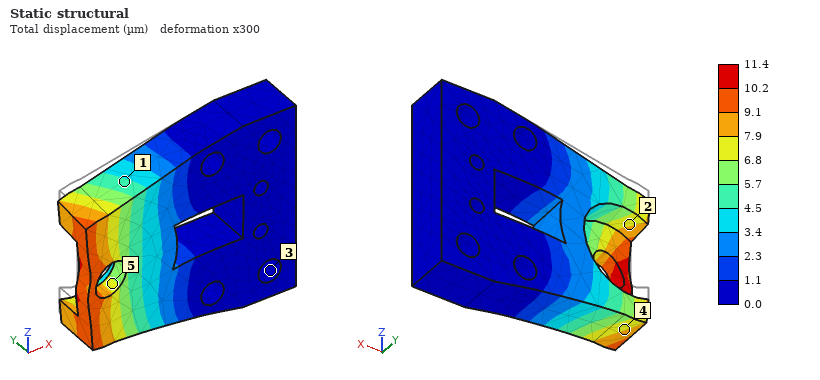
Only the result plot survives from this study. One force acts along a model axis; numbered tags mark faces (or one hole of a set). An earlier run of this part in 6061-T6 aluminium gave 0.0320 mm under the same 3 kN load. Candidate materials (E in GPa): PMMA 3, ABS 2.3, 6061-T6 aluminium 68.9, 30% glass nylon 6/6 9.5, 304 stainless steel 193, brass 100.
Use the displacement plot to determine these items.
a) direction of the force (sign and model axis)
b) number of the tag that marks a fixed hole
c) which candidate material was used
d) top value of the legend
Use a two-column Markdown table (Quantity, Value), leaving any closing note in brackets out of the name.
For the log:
| Quantity | Value |
|---|---|
| direction of the force | -Z |
| number of the tag that marks a fixed hole | 3 |
| which candidate material was used | 304 stainless steel |
| top value of the legend | 11.4 µm |
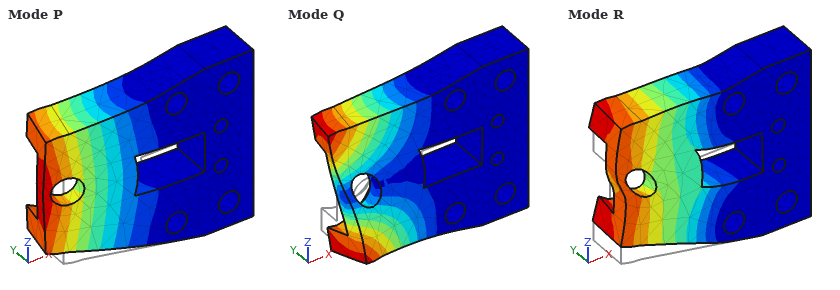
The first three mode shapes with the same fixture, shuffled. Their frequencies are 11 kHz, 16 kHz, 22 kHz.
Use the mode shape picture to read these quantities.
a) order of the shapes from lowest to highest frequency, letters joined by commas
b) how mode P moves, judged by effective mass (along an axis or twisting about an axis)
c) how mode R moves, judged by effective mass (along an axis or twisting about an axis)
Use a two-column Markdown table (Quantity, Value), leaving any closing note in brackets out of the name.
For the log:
| Quantity | Value |
|---|---|
| order of the shapes from lowest to highest frequency, letters joined by commas | P, Q, R |
| how mode P moves, judged by effective mass | along Y |
| how mode R moves, judged by effective mass | along Z |
